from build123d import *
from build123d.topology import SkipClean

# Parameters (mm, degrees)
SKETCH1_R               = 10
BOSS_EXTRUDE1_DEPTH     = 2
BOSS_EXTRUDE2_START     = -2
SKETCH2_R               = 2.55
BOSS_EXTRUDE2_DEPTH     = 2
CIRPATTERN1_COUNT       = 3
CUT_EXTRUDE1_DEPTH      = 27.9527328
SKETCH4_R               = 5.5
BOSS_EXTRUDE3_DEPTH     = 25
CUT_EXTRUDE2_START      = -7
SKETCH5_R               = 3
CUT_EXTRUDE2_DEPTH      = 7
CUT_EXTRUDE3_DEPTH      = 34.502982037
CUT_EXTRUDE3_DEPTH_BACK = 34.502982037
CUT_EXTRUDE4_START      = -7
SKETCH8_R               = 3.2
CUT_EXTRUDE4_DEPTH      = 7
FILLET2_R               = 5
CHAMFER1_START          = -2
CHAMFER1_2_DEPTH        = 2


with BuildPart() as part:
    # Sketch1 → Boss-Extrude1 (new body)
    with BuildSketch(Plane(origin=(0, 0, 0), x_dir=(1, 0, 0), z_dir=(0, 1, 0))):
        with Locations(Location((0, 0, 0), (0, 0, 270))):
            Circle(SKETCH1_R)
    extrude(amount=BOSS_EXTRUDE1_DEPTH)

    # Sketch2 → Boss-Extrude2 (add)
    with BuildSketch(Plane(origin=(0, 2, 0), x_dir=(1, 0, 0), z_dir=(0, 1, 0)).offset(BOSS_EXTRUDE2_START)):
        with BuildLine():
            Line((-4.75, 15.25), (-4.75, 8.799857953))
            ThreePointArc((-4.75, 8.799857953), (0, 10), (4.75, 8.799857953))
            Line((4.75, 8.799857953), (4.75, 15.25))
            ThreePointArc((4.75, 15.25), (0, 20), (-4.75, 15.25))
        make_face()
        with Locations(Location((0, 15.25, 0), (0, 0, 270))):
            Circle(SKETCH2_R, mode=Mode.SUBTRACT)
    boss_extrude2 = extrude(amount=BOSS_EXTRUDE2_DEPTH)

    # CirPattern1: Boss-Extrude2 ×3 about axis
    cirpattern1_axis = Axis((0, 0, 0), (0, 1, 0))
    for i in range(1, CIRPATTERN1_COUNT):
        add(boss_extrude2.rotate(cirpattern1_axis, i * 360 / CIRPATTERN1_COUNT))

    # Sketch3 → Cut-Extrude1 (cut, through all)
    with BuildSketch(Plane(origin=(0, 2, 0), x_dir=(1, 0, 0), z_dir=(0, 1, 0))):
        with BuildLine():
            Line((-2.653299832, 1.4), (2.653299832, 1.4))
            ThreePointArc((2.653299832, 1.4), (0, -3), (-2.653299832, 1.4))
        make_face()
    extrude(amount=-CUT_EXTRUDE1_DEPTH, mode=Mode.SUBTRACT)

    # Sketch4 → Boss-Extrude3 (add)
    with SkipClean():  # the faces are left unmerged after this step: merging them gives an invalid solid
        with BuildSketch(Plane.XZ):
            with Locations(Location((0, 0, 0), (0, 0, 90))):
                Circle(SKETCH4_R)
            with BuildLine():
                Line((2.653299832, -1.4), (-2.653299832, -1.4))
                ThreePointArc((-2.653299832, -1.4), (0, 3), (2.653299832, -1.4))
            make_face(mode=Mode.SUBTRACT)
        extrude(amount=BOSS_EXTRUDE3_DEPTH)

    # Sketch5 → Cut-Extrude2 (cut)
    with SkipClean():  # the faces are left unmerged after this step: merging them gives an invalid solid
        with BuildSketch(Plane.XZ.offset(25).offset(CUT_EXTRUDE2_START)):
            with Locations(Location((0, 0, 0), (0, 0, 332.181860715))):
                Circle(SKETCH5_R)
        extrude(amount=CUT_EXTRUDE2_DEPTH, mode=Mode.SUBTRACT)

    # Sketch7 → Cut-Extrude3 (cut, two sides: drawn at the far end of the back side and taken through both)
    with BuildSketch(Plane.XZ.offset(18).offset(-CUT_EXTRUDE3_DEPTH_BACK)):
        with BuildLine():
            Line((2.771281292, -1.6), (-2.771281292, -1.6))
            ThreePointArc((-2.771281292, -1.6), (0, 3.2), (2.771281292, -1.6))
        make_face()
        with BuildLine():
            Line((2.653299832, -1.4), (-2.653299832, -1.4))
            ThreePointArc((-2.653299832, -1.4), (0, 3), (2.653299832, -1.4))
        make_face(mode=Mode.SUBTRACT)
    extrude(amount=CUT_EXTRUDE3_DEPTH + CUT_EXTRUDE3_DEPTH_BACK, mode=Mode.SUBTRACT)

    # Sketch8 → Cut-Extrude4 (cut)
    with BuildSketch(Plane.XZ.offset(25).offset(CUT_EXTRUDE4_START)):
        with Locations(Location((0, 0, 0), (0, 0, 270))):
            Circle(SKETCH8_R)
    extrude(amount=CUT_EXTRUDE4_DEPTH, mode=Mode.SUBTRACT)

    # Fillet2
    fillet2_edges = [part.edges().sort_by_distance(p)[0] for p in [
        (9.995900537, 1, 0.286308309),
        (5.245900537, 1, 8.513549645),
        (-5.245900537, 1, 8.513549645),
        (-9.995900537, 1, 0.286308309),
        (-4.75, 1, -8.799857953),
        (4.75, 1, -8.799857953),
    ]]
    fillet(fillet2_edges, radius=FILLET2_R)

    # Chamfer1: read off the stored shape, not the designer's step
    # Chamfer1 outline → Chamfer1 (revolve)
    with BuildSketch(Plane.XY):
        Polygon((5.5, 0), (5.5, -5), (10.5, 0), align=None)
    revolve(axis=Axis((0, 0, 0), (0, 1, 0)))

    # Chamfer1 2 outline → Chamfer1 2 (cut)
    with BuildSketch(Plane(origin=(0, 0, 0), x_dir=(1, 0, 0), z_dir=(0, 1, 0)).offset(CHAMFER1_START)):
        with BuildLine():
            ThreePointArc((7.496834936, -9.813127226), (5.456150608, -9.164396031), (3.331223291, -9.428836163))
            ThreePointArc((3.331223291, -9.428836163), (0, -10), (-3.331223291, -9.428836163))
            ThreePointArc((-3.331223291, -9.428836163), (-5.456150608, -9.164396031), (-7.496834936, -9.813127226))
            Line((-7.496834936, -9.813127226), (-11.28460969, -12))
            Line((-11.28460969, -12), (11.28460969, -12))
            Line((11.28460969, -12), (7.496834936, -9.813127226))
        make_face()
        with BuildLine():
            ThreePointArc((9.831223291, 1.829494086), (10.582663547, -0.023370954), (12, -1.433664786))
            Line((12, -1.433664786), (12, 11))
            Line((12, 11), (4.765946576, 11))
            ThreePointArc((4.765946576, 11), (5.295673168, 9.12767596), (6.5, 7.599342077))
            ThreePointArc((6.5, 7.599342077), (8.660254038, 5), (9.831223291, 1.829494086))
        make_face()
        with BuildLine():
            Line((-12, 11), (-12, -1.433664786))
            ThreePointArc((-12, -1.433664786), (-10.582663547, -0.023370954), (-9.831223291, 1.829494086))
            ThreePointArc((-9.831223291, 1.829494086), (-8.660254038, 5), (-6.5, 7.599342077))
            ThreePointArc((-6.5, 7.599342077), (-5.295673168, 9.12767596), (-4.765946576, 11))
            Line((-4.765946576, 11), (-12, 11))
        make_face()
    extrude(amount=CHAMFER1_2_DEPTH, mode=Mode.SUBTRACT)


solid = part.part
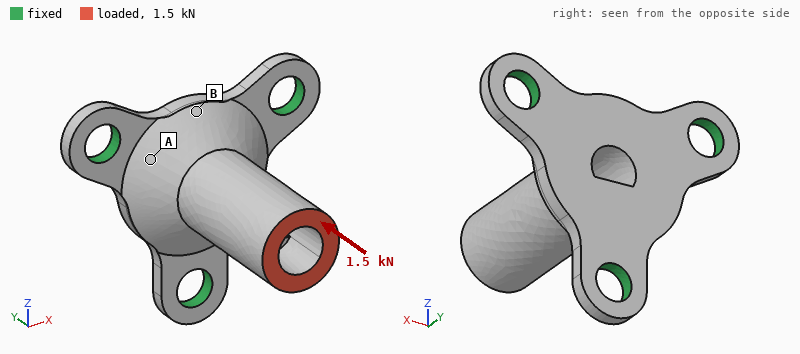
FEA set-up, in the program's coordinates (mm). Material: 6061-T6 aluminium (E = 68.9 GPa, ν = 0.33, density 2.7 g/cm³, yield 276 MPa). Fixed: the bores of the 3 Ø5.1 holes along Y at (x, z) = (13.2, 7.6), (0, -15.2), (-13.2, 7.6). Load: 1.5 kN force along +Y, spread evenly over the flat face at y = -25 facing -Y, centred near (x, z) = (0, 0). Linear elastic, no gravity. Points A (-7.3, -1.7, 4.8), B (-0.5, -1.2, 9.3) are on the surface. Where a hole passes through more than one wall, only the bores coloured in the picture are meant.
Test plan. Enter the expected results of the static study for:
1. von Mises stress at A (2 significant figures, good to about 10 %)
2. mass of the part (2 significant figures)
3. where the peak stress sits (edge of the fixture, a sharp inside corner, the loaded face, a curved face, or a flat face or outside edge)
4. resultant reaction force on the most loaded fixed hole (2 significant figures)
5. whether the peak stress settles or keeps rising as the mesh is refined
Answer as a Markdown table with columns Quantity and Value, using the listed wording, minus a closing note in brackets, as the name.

| Quantity | Value |
|---|---|
| von Mises stress at A | 77 MPa |
| mass of the part | 8.8 g |
| where the peak stress sits | edge of the fixture |
| resultant reaction force on the most loaded fixed hole | 670 N |
| whether the peak stress settles or keeps rising as the mesh is refined | keeps rising |
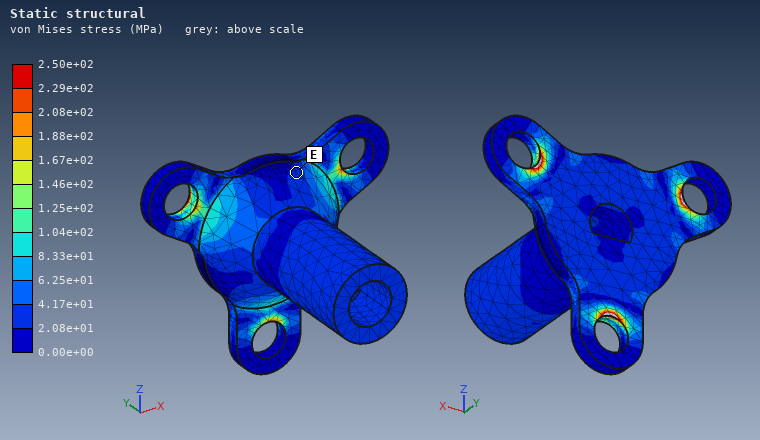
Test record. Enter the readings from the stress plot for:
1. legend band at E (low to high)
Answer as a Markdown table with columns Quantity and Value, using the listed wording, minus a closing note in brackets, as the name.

| Quantity | Value |
|---|---|
| legend band at E | 2.08e+01 to 4.17e+01 MPa |
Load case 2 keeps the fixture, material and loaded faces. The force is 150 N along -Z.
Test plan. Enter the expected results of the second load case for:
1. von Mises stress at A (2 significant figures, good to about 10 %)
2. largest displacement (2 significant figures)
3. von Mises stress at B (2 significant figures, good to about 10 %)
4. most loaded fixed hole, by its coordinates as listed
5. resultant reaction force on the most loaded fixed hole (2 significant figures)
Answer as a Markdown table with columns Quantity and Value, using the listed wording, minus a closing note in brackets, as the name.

| Quantity | Value |
|---|---|
| von Mises stress at A | 20 MPa |
| largest displacement | 36 µm |
| von Mises stress at B | 5.9 MPa |
| most loaded fixed hole, by its coordinates as listed | (0, -15.2) |
| resultant reaction force on the most loaded fixed hole | 250 N |
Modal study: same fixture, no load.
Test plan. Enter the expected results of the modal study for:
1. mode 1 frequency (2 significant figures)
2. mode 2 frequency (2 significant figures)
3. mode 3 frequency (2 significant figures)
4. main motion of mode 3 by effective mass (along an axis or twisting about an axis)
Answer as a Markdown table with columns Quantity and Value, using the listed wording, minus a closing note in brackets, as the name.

| Quantity | Value |
|---|---|
| mode 1 frequency | 9000 Hz |
| mode 2 frequency | 9000 Hz |
| mode 3 frequency | 16 kHz |
| main motion of mode 3 by effective mass | along Y |
